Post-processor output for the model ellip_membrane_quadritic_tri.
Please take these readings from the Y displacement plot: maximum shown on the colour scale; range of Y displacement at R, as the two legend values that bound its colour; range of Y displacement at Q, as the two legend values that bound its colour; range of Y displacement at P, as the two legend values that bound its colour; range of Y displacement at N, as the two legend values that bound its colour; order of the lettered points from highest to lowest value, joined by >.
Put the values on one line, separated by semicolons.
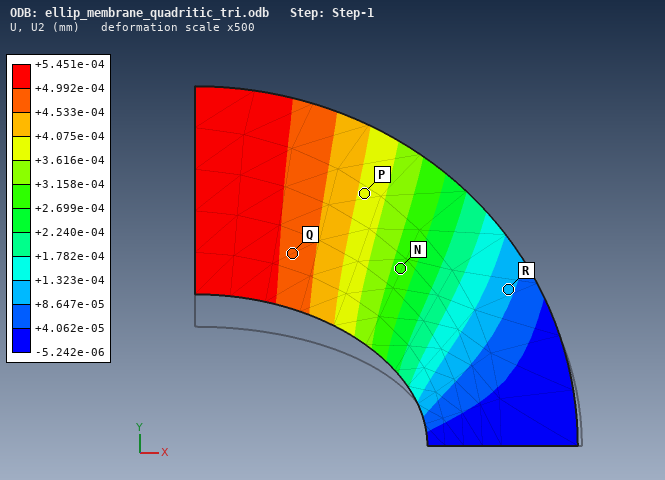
+5.451e-04 mm; +8.647e-05 to +1.323e-04 mm; +4.533e-04 to +4.992e-04 mm; +3.616e-04 to +4.075e-04 mm; +2.699e-04 to +3.158e-04 mm; Q > P > N > R
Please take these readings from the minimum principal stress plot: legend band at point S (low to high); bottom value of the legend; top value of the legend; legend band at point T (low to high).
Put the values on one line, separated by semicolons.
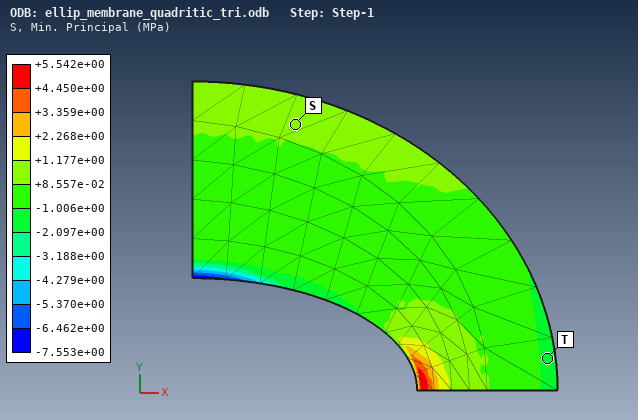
+8.557e-02 to +1.177e+00 MPa; -7.553e+00 MPa; +5.542e+00 MPa; -2.097e+00 to -1.006e+00 MPa
